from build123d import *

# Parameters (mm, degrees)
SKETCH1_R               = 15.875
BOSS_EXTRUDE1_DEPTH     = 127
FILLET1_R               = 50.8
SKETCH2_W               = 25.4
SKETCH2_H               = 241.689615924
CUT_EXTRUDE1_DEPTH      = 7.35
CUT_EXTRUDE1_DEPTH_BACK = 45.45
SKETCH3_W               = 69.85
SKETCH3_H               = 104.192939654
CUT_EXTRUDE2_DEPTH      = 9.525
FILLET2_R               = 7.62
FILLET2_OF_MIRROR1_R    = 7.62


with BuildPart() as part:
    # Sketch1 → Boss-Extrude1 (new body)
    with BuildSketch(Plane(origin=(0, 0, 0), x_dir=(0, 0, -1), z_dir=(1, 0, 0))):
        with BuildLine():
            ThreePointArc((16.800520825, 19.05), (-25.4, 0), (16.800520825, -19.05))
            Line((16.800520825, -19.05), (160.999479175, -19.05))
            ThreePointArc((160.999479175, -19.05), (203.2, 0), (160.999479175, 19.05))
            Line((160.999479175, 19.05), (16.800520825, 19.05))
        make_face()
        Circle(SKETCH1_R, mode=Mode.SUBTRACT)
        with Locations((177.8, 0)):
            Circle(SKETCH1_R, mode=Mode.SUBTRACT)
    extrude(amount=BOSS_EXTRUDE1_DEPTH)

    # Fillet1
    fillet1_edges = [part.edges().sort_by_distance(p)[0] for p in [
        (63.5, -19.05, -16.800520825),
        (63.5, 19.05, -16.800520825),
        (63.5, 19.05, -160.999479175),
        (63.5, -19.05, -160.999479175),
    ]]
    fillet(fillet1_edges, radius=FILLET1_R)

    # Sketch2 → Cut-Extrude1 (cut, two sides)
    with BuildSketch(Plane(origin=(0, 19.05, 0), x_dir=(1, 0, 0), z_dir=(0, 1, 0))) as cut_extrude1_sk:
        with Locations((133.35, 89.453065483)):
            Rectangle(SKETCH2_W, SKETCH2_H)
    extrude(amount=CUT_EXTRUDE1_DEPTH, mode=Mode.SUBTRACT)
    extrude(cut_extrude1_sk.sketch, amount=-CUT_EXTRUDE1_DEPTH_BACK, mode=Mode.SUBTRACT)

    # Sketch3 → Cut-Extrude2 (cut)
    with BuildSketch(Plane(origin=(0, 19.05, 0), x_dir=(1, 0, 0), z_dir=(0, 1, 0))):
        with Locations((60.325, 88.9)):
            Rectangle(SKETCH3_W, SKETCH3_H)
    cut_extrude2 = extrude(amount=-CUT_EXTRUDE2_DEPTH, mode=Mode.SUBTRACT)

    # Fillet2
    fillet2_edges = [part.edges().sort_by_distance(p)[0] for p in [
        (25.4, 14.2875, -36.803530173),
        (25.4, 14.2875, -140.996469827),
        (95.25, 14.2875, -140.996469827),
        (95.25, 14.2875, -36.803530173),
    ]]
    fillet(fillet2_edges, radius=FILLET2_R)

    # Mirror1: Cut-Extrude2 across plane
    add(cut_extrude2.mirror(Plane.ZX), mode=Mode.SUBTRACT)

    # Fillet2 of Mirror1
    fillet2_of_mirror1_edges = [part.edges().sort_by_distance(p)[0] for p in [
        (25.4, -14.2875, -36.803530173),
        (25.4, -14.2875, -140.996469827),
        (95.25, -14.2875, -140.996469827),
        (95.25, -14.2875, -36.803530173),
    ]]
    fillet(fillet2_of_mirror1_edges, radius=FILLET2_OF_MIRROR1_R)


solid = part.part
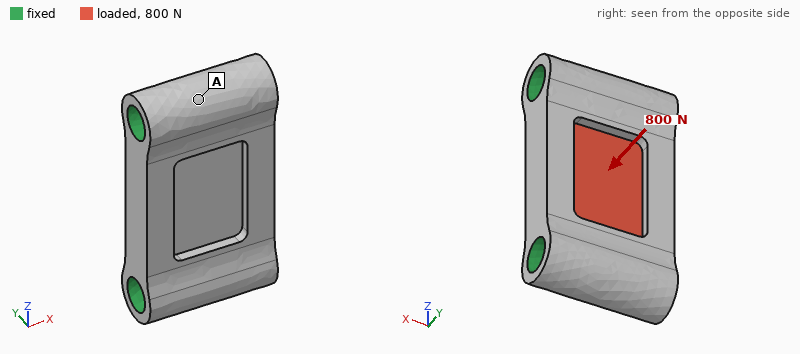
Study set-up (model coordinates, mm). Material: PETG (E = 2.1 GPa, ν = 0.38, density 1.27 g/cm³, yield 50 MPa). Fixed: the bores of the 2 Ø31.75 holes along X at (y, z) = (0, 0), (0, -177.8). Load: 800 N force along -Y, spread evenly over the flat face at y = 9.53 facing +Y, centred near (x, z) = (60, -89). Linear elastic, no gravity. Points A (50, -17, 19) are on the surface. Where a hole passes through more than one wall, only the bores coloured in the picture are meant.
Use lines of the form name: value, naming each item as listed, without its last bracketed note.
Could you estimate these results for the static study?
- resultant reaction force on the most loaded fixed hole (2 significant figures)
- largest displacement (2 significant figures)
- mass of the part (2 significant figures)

resultant reaction force on the most loaded fixed hole: 400 N
largest displacement: 32 µm
mass of the part: 980 g
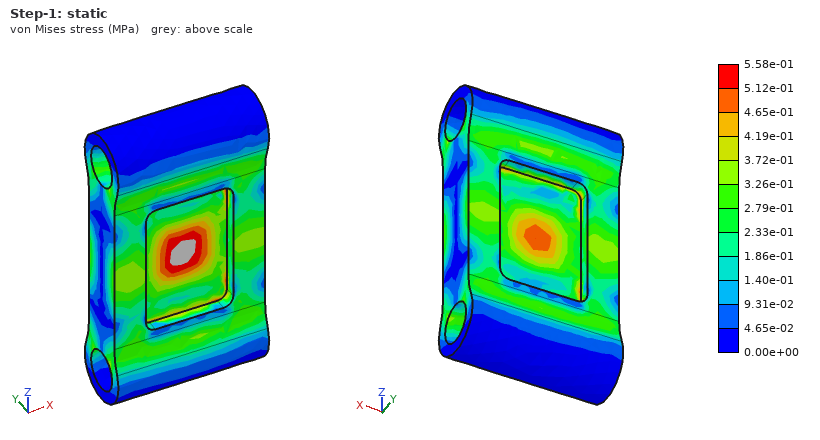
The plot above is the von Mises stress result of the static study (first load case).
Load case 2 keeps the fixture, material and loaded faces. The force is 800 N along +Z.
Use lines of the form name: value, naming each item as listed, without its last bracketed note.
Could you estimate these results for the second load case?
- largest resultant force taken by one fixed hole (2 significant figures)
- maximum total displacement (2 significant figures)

largest resultant force taken by one fixed hole: 400 N
maximum total displacement: 5.6 µm
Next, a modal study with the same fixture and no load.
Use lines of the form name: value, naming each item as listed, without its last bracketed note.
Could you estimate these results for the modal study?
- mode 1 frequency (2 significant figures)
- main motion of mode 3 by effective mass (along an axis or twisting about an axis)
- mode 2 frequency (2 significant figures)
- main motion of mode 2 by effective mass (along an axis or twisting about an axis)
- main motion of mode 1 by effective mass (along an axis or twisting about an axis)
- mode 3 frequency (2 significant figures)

mode 1 frequency: 1600 Hz
main motion of mode 3 by effective mass: along X
mode 2 frequency: 1800 Hz
main motion of mode 2 by effective mass: twisting about Z
main motion of mode 1 by effective mass: along Y
mode 3 frequency: 2300 Hz
